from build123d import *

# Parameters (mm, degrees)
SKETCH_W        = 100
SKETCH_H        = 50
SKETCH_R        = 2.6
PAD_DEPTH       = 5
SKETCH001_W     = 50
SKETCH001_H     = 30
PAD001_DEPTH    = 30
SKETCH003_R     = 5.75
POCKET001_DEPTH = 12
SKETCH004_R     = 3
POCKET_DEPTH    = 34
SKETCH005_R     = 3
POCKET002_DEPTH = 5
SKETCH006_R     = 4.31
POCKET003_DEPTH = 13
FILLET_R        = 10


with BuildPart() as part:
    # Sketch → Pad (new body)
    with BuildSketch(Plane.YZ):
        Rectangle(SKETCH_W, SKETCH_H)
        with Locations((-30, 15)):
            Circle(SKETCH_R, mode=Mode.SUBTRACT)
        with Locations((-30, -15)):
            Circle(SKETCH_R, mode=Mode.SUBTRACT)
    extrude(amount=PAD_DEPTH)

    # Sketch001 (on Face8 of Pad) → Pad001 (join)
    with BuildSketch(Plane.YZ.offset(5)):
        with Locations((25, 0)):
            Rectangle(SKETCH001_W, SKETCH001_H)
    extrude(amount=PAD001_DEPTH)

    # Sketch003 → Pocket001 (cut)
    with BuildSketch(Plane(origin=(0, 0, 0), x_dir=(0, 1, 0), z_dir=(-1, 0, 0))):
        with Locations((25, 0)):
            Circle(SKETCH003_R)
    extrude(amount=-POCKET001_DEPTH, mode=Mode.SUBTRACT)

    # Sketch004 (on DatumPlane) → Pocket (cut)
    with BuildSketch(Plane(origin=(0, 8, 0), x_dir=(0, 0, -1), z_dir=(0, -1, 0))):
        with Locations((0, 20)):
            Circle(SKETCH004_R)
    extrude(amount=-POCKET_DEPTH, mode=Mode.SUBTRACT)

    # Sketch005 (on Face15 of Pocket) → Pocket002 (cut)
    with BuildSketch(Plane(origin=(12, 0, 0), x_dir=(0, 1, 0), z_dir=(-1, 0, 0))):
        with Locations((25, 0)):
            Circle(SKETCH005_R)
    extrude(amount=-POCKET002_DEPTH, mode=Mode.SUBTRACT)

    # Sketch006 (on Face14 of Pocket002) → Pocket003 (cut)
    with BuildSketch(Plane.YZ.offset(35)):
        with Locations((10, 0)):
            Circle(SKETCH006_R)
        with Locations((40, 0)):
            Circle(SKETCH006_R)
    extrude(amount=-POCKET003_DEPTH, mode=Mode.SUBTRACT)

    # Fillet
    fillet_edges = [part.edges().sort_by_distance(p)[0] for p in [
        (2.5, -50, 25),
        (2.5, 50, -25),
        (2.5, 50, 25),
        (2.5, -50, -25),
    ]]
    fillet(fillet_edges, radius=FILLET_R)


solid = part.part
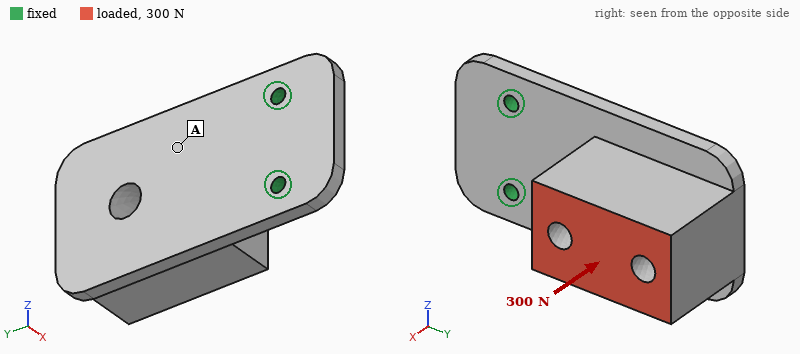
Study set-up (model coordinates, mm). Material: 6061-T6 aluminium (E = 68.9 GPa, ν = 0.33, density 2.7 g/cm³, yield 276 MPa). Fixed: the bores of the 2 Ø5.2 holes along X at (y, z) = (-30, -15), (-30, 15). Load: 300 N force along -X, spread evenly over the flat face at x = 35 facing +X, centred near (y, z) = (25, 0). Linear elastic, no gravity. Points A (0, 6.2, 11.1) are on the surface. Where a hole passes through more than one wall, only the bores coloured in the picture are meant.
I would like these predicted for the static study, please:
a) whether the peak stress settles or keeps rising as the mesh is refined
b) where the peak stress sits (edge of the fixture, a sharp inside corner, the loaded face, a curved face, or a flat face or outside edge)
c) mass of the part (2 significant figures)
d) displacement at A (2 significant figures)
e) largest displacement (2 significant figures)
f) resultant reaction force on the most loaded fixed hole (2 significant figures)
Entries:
keeps rising
edge of the fixture
180 g
0.23 mm
0.75 mm
150 N
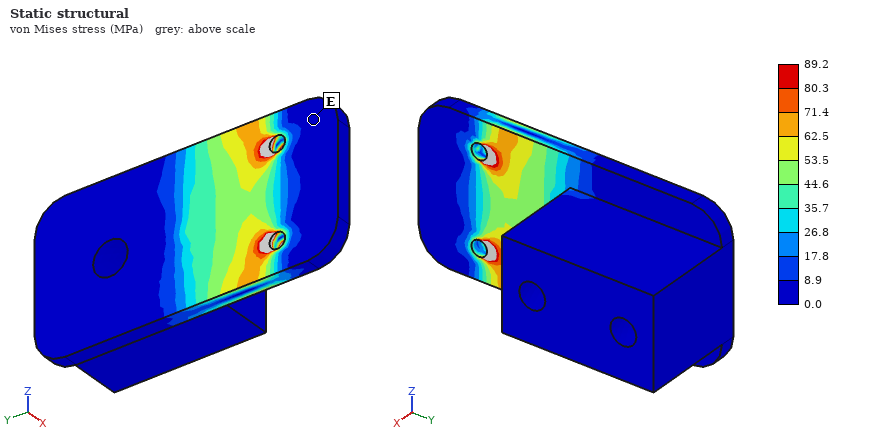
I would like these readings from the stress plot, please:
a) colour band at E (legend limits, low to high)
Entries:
0.0 to 8.9 MPa
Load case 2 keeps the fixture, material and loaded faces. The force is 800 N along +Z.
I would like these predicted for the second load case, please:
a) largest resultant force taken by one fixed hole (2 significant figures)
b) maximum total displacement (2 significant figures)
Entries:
1.6 kN
0.29 mm
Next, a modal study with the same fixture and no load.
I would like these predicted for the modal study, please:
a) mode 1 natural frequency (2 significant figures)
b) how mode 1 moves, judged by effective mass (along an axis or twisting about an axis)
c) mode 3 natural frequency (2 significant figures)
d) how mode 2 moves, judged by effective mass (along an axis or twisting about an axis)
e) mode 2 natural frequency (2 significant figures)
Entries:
310 Hz
along X
2600 Hz
along Z
1200 Hz
